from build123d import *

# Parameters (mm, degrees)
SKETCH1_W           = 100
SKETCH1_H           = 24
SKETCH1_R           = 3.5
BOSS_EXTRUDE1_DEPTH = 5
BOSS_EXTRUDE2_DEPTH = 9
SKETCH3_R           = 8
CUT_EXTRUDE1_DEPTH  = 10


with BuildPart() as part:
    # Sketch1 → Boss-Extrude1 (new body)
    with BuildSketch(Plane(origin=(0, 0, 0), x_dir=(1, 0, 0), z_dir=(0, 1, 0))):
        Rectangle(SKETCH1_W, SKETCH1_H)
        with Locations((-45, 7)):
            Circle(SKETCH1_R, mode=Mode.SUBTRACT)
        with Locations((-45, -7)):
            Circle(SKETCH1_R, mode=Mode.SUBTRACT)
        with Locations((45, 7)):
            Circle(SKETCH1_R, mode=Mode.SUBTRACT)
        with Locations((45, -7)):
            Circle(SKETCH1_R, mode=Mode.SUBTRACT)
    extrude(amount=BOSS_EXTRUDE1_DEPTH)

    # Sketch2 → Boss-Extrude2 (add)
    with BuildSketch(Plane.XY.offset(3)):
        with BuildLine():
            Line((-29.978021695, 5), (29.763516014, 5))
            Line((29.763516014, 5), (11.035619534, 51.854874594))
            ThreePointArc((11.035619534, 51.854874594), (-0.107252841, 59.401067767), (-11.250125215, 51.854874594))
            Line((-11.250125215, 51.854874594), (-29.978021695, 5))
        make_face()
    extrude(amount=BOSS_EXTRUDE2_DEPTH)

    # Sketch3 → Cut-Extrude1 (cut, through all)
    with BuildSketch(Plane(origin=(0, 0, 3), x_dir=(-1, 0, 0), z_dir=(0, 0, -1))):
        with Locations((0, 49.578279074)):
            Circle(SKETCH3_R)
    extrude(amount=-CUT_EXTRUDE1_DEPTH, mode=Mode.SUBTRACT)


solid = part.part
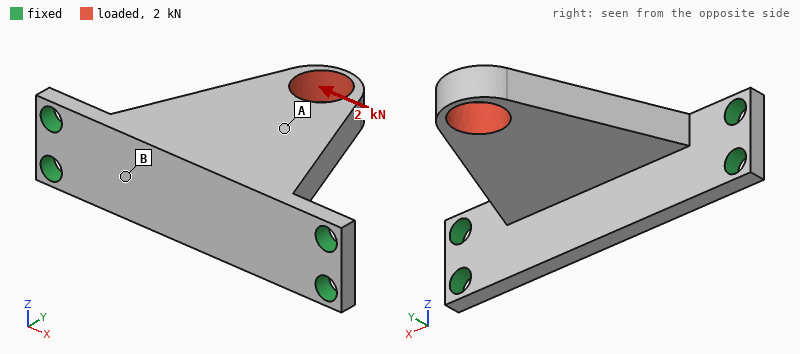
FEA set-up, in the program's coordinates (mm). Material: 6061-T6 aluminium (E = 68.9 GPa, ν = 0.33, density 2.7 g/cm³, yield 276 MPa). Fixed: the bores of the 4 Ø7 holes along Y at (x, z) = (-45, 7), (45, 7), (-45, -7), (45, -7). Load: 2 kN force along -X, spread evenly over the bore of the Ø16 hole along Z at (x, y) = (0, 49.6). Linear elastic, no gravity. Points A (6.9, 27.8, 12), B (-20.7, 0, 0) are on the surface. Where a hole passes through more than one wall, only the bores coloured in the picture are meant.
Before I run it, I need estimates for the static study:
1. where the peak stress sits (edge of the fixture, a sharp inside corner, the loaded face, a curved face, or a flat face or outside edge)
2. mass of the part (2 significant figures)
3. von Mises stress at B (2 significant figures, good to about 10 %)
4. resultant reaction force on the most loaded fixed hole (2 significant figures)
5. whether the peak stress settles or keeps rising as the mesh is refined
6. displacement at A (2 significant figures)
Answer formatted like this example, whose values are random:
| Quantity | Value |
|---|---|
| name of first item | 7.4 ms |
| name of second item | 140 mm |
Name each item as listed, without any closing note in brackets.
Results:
| Quantity | Value |
|---|---|
| where the peak stress sits | edge of the fixture |
| mass of the part | 75 g |
| von Mises stress at B | 30 MPa |
| resultant reaction force on the most loaded fixed hole | 1.3 kN |
| whether the peak stress settles or keeps rising as the mesh is refined | keeps rising |
| displacement at A | 0.044 mm |
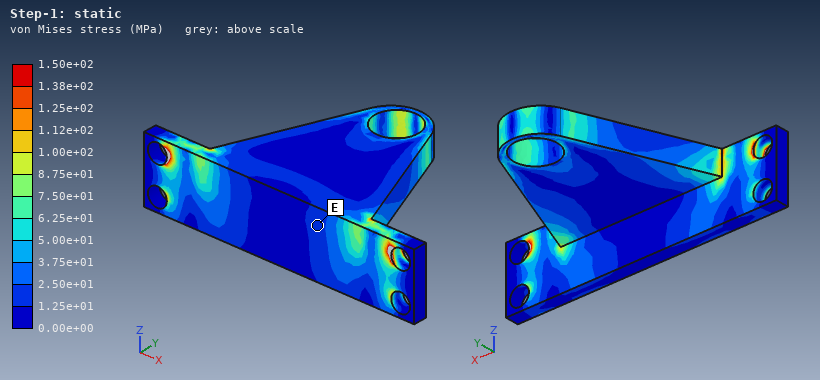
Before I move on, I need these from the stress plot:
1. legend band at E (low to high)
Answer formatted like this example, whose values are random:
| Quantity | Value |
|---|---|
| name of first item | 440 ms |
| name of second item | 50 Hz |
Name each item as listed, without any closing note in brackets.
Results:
| Quantity | Value |
|---|---|
| legend band at E | 1.25e+01 to 2.50e+01 MPa |
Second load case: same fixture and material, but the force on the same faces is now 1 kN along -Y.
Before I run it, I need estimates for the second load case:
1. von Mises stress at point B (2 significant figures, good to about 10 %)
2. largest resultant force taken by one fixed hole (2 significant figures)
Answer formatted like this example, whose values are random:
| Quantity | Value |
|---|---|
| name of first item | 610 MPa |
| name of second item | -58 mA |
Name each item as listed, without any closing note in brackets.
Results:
| Quantity | Value |
|---|---|
| von Mises stress at point B | 7.3 MPa |
| largest resultant force taken by one fixed hole | 570 N |
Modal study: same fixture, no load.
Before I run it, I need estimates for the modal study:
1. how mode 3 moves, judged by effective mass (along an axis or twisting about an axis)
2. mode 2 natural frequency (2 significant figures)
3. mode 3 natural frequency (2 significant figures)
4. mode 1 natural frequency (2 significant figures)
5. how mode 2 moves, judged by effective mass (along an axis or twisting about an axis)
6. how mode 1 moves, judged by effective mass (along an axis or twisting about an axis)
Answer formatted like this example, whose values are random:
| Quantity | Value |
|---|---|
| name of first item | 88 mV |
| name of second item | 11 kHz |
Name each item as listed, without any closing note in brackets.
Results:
| Quantity | Value |
|---|---|
| how mode 3 moves, judged by effective mass | along X |
| mode 2 natural frequency | 4300 Hz |
| mode 3 natural frequency | 5700 Hz |
| mode 1 natural frequency | 1500 Hz |
| how mode 2 moves, judged by effective mass | along Y |
| how mode 1 moves, judged by effective mass | along Z |
